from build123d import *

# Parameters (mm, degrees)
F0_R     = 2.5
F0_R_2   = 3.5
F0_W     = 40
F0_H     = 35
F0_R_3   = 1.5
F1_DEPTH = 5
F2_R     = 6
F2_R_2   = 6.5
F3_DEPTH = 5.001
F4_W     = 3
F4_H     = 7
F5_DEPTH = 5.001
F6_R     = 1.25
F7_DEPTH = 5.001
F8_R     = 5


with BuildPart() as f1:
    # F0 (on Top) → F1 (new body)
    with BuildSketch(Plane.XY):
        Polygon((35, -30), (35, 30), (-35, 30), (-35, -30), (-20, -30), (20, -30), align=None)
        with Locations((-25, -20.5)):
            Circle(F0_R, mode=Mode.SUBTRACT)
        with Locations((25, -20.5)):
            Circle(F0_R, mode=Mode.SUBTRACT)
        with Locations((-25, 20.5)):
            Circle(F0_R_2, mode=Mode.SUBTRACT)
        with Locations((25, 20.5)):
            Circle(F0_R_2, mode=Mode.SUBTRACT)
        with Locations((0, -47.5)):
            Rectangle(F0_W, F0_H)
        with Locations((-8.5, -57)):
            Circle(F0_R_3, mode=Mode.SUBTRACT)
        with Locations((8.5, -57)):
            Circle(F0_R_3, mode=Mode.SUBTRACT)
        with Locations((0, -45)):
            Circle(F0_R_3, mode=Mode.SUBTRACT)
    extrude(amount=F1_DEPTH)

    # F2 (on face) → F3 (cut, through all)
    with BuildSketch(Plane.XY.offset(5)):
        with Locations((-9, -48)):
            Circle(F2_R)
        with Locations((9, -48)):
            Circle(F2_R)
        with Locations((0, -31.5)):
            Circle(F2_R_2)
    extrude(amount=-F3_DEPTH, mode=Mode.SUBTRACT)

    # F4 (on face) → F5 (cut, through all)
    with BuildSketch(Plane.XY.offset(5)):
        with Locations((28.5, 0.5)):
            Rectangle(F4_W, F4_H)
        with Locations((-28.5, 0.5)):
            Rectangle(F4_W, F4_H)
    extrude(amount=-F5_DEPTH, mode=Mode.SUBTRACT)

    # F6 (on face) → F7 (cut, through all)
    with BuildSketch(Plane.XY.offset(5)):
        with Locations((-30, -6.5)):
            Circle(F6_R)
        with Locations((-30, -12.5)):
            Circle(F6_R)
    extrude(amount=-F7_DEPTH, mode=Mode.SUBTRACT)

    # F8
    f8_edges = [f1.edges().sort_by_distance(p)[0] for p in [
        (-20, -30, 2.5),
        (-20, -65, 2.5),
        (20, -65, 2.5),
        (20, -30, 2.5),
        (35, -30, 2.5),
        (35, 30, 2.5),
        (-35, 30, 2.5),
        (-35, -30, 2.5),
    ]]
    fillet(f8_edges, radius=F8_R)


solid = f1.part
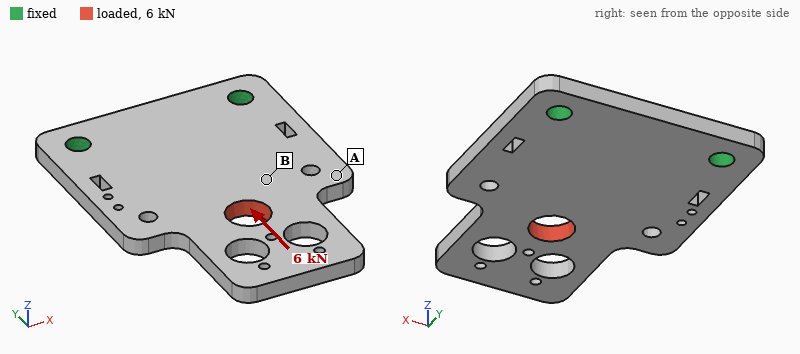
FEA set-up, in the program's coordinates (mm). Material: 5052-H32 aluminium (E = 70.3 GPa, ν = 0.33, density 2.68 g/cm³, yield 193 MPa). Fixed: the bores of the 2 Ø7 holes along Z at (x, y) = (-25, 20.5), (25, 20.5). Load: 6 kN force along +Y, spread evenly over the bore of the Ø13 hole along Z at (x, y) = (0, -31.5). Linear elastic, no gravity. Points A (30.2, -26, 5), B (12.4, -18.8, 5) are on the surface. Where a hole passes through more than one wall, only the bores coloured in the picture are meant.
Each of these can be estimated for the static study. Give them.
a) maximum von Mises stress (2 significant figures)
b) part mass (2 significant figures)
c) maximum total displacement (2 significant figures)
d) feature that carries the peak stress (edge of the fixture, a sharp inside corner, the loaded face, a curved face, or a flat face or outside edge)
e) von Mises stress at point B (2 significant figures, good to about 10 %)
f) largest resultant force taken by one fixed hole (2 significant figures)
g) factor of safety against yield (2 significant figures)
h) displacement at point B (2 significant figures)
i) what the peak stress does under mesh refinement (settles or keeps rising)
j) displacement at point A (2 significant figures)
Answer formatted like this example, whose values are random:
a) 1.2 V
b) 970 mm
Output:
a) 78 MPa
b) 67 g
c) 30 µm
d) a curved face
e) 27 MPa
f) 3.1 kN
g) 2.5
h) 15 µm
i) settles
j) 9.8 µm
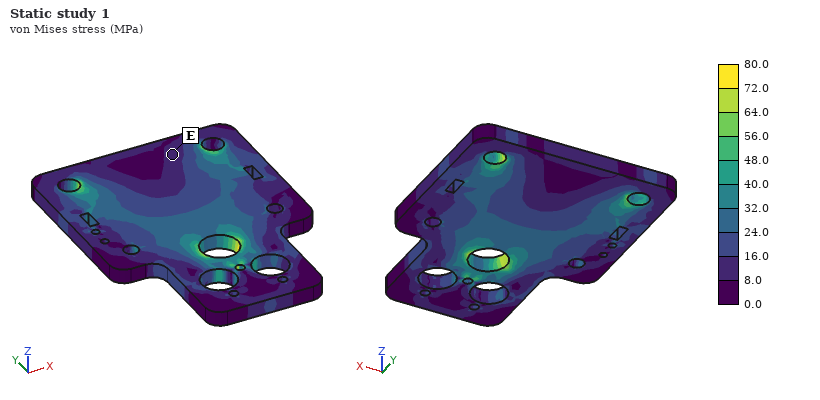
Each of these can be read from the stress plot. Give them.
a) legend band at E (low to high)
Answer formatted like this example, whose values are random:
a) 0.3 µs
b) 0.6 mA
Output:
a) 8.0 to 16.0 MPa
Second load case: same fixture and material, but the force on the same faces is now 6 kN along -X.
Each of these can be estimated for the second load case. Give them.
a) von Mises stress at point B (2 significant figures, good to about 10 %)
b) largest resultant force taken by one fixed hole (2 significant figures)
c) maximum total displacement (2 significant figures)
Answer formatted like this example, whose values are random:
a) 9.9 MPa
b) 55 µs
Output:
a) 33 MPa
b) 6.5 kN
c) 0.11 mm
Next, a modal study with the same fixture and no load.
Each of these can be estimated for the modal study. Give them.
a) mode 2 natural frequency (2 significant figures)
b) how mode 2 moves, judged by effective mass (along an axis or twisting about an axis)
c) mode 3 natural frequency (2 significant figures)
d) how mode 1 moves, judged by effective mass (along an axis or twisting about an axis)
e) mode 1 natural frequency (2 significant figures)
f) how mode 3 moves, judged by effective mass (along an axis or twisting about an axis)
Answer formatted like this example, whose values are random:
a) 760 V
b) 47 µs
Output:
a) 2600 Hz
b) twisting about Y
c) 3100 Hz
d) along Z
e) 750 Hz
f) along Z
